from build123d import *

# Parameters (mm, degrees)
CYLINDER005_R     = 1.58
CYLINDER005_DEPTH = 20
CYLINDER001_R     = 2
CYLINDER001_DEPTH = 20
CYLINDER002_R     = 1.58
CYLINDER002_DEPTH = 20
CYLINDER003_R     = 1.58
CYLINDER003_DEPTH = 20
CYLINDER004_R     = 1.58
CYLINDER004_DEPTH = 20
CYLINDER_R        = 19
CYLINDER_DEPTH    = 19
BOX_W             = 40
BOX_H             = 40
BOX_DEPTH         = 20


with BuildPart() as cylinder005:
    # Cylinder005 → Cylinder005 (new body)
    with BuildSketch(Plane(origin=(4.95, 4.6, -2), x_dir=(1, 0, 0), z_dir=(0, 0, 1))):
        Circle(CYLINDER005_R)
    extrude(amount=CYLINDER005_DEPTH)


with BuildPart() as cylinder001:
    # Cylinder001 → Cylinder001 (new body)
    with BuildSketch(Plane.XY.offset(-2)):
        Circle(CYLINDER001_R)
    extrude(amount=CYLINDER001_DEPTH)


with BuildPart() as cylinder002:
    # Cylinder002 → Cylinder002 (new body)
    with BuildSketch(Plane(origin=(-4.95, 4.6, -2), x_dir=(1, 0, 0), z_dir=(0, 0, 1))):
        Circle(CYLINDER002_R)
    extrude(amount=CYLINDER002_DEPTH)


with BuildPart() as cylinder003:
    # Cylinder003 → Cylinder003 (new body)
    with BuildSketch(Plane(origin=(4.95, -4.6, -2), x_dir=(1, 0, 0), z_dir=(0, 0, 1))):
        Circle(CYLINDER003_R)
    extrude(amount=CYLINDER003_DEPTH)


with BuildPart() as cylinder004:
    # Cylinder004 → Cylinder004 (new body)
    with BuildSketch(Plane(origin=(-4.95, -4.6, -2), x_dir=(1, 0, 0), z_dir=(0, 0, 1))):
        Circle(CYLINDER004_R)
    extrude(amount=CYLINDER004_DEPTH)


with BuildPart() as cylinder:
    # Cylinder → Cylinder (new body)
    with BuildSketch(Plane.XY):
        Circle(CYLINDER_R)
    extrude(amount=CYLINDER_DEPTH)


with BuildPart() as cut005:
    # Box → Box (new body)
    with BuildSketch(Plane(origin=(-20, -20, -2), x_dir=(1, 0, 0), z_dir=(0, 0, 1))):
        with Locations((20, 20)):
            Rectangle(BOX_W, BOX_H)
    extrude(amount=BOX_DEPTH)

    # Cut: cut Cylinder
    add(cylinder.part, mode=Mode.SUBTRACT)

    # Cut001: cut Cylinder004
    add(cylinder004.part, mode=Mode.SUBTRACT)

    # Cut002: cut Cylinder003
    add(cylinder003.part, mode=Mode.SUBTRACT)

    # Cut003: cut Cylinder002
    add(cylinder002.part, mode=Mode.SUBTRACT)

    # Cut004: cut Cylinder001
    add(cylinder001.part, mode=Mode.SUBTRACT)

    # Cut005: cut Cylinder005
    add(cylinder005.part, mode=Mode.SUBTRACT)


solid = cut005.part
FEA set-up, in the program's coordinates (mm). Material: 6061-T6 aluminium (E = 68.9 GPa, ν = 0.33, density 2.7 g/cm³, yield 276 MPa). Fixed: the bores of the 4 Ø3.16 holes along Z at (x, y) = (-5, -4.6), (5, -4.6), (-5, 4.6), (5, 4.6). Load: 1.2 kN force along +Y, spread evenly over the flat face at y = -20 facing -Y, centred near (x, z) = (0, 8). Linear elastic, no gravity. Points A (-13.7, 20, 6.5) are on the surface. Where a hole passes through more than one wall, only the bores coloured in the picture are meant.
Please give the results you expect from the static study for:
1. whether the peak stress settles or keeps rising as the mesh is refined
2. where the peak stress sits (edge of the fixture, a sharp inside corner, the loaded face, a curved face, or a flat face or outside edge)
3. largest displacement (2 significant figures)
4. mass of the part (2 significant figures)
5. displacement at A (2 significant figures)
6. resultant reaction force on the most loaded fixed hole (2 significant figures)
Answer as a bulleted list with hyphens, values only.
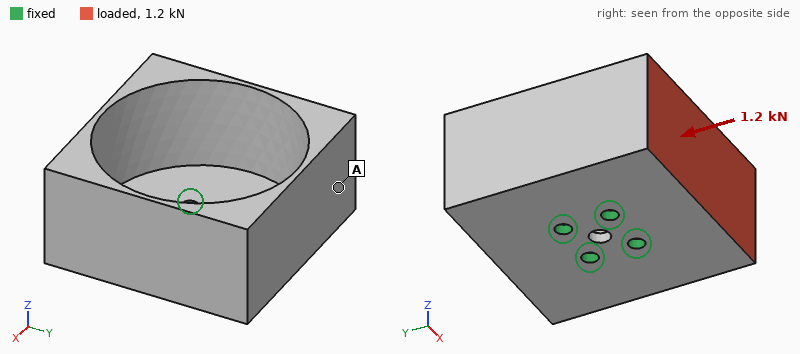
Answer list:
- keeps rising
- edge of the fixture
- 0.20 mm
- 31 g
- 0.12 mm
- 550 N
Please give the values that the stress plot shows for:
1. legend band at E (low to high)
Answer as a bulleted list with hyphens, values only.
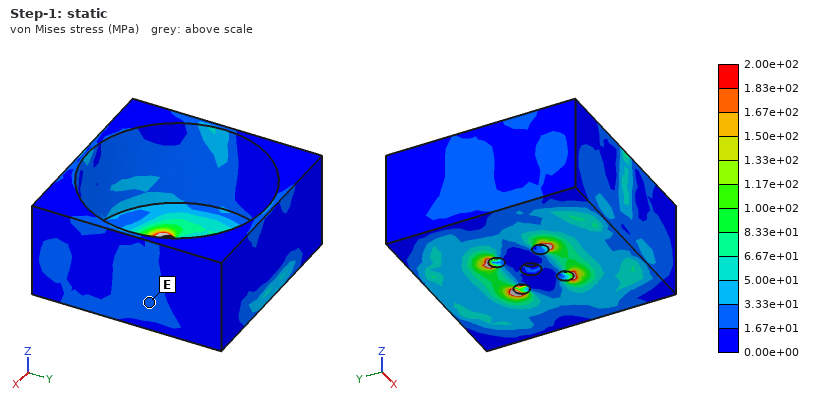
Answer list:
- 1.67e+01 to 3.33e+01 MPa
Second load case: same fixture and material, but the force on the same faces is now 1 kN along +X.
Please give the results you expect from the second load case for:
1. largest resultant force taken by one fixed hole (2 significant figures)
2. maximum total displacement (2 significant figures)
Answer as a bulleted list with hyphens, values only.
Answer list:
- 940 N
- 0.21 mm
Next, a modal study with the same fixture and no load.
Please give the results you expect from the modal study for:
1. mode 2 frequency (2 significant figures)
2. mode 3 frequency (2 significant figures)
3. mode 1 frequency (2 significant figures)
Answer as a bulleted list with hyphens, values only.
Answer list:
- 2400 Hz
- 3300 Hz
- 2300 Hz
